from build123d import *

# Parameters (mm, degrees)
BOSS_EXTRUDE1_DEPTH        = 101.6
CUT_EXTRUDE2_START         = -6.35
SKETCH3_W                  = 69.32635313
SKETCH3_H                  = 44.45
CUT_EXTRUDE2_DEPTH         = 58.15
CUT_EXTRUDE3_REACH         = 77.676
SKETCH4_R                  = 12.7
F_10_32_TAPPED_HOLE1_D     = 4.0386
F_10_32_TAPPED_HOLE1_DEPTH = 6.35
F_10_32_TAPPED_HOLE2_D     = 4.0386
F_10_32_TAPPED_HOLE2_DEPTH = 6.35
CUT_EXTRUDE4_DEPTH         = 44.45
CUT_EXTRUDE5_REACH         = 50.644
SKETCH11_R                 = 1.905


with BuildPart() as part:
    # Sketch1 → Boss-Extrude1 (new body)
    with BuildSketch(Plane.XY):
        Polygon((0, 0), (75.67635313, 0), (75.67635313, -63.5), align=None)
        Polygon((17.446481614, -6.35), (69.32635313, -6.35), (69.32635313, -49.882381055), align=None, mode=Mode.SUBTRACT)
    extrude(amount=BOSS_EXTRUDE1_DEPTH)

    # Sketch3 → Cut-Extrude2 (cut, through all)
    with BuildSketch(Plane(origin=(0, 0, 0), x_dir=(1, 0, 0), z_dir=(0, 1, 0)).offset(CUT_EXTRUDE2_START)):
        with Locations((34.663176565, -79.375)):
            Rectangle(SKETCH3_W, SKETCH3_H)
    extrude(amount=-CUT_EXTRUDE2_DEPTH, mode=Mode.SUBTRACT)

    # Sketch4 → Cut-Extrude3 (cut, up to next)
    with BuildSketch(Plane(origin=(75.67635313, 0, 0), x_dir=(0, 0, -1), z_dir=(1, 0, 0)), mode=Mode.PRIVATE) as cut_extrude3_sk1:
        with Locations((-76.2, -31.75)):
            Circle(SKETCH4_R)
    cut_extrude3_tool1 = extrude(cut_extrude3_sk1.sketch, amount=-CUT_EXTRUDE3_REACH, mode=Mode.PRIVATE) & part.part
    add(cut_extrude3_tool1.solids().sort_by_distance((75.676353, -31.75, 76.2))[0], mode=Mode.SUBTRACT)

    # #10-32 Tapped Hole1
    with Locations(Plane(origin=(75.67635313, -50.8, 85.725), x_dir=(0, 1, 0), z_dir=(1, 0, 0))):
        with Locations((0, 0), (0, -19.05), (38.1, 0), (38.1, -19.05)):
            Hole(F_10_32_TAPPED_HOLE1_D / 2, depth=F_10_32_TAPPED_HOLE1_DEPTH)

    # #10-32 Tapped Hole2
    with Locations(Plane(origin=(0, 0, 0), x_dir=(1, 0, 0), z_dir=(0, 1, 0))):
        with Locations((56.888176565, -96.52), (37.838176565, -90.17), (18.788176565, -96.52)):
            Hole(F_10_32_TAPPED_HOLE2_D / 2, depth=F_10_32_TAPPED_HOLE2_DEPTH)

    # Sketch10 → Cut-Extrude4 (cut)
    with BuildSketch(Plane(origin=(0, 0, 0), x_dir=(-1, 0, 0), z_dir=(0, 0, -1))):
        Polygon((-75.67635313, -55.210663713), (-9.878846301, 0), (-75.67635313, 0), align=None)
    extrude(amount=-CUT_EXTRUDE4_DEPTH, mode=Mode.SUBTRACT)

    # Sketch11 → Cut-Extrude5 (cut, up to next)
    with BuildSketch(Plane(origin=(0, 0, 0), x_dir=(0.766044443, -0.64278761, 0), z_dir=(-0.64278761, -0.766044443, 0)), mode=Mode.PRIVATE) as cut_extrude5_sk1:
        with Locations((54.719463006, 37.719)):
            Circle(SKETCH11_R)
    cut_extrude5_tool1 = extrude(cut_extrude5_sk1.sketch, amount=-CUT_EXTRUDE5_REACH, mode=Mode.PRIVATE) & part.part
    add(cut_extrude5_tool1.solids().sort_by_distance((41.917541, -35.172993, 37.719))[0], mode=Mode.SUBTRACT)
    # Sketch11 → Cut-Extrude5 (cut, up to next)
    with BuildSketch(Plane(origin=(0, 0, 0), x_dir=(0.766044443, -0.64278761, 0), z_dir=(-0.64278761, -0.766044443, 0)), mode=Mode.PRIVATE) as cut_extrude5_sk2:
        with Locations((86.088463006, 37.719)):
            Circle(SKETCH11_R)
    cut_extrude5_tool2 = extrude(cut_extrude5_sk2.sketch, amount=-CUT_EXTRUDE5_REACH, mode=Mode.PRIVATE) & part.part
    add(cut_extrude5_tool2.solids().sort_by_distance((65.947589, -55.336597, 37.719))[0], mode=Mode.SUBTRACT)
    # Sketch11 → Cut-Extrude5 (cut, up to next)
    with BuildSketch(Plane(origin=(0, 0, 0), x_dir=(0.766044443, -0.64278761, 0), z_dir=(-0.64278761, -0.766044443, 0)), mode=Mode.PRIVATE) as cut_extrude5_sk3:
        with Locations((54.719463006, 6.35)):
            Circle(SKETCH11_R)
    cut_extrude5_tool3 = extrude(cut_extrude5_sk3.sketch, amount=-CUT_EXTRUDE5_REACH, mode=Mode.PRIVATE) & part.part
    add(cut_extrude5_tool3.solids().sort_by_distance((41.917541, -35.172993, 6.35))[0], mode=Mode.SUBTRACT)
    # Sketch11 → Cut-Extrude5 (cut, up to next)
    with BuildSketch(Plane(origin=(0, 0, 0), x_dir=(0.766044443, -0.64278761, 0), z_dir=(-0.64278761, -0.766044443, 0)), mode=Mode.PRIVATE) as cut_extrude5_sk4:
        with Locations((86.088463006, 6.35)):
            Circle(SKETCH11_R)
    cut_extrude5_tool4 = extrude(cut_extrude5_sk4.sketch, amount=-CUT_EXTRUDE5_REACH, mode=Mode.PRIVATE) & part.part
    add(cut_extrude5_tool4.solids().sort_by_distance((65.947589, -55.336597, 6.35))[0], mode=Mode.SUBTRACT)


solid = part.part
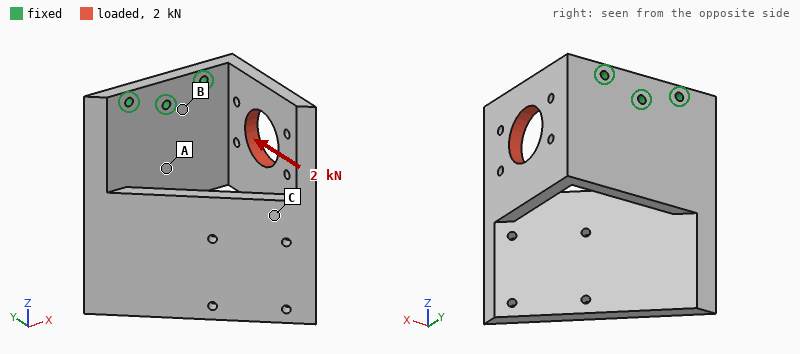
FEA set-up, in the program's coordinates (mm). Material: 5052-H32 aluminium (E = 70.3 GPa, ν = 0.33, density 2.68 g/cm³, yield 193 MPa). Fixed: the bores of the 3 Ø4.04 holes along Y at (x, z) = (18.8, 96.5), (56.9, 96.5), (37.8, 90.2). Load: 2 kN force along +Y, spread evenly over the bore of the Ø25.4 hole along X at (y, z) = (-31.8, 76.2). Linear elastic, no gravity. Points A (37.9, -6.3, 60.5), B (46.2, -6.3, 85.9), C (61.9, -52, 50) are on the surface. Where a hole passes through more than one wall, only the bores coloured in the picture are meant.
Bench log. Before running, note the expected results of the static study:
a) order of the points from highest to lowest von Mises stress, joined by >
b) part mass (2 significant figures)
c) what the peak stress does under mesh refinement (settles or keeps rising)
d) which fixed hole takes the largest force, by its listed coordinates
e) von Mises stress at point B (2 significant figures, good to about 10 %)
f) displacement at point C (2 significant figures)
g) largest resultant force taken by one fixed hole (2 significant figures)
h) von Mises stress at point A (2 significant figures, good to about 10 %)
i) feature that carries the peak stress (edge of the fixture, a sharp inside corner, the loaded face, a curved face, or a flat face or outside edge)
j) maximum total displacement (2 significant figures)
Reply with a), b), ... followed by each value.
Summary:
a) B > A > C
b) 200 g
c) keeps rising
d) (56.9, 96.5)
e) 78 MPa
f) 0.47 mm
g) 2.0 kN
h) 26 MPa
i) edge of the fixture
j) 0.79 mm
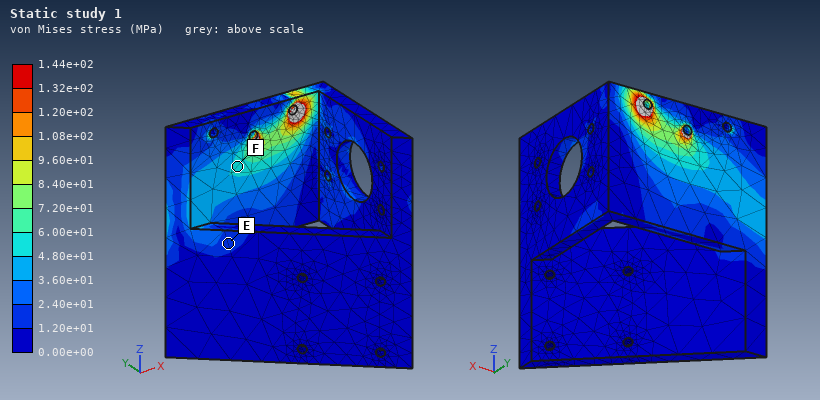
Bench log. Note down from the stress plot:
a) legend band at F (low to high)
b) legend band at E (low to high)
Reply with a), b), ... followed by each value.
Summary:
a) 4.80e+01 to 6.00e+01 MPa
b) 1.20e+01 to 2.40e+01 MPa
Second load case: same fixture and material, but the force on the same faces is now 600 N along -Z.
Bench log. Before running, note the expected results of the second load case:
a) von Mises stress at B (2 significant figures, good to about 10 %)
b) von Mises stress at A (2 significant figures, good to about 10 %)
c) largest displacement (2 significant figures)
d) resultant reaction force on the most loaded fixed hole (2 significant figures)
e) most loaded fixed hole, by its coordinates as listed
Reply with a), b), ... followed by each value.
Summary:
a) 29 MPa
b) 8.6 MPa
c) 0.35 mm
d) 750 N
e) (56.9, 96.5)
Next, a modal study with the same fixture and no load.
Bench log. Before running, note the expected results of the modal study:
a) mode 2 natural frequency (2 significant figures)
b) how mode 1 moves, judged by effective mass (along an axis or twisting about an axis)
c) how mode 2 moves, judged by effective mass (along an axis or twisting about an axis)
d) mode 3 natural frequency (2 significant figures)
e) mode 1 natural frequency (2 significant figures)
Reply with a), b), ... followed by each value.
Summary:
a) 1100 Hz
b) along Y
c) along X
d) 1600 Hz
e) 520 Hz
